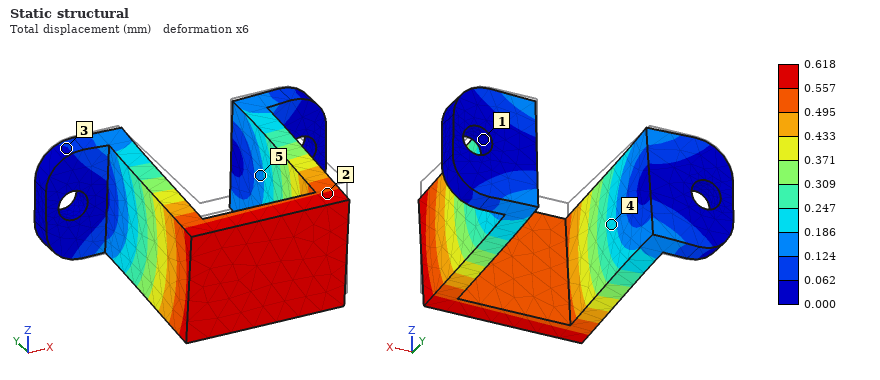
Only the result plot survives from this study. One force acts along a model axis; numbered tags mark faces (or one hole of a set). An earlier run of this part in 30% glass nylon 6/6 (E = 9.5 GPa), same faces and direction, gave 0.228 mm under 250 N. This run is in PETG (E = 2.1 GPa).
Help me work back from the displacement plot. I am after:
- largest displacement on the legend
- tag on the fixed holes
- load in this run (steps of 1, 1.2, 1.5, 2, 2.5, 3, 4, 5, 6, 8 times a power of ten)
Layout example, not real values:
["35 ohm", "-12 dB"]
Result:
["0.618 mm", "1", "150 N"]
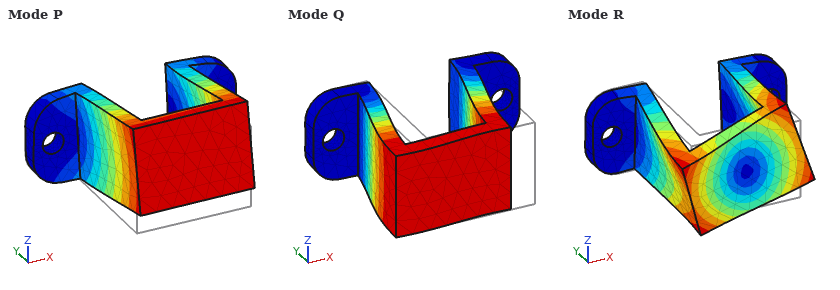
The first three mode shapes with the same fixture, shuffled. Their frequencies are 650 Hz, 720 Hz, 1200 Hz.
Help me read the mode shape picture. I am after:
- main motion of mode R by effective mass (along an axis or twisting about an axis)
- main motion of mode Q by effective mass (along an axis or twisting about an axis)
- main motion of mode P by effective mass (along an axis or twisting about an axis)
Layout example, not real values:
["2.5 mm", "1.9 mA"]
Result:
["twisting about Y", "along X", "along Z"]
